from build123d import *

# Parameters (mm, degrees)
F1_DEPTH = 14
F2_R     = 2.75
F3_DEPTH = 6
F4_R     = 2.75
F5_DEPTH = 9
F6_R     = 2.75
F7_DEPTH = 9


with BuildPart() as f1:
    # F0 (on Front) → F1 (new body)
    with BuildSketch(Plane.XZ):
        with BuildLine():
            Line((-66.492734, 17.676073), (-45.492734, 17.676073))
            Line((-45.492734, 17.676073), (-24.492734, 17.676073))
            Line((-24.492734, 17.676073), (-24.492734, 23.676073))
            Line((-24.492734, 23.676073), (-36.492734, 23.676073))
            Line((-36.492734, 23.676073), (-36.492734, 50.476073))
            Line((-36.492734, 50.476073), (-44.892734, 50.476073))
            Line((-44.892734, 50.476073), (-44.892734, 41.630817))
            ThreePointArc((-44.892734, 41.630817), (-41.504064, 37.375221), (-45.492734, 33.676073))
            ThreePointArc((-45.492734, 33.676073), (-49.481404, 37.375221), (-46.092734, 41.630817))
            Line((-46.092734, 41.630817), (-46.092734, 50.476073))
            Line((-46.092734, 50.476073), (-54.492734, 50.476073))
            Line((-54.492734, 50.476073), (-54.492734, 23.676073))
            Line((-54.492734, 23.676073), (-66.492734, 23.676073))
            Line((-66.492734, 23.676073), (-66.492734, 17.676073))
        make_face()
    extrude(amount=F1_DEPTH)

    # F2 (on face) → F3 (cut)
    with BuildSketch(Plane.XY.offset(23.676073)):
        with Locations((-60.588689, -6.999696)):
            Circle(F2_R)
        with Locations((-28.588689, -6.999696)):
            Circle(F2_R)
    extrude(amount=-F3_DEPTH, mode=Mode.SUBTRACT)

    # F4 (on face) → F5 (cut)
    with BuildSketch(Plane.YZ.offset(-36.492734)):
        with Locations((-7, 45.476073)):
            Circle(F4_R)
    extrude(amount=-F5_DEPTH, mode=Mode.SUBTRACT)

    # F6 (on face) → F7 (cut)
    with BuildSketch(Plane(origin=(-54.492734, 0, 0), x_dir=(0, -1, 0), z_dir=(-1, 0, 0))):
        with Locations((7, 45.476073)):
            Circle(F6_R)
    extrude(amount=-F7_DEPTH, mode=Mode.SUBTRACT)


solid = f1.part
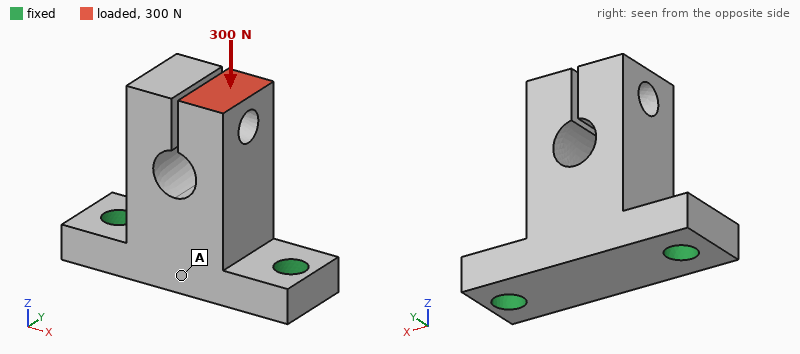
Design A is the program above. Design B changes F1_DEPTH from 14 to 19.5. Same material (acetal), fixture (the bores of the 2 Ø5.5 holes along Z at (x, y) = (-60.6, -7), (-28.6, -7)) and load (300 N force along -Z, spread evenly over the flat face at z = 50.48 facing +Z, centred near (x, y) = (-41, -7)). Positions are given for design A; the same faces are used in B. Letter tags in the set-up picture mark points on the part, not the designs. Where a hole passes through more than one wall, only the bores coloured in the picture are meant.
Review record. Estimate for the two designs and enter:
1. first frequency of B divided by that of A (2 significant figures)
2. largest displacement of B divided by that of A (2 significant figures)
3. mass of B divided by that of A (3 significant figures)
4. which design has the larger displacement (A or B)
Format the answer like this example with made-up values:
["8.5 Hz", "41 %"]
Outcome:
["0.97", "0.89", "1.42", "A"]
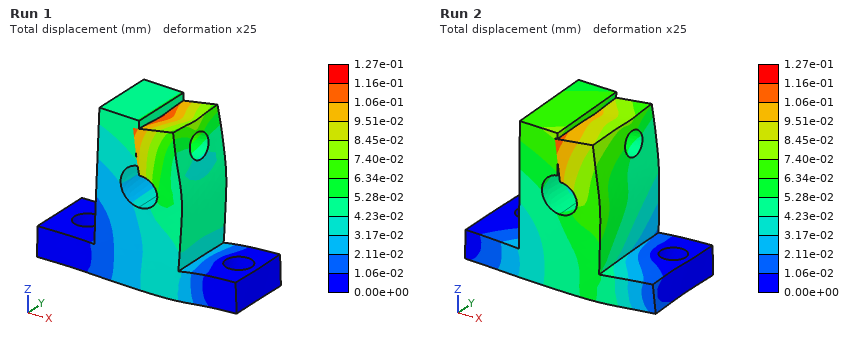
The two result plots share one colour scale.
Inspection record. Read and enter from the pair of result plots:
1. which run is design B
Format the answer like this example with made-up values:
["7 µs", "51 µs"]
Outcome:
["Run 2"]
